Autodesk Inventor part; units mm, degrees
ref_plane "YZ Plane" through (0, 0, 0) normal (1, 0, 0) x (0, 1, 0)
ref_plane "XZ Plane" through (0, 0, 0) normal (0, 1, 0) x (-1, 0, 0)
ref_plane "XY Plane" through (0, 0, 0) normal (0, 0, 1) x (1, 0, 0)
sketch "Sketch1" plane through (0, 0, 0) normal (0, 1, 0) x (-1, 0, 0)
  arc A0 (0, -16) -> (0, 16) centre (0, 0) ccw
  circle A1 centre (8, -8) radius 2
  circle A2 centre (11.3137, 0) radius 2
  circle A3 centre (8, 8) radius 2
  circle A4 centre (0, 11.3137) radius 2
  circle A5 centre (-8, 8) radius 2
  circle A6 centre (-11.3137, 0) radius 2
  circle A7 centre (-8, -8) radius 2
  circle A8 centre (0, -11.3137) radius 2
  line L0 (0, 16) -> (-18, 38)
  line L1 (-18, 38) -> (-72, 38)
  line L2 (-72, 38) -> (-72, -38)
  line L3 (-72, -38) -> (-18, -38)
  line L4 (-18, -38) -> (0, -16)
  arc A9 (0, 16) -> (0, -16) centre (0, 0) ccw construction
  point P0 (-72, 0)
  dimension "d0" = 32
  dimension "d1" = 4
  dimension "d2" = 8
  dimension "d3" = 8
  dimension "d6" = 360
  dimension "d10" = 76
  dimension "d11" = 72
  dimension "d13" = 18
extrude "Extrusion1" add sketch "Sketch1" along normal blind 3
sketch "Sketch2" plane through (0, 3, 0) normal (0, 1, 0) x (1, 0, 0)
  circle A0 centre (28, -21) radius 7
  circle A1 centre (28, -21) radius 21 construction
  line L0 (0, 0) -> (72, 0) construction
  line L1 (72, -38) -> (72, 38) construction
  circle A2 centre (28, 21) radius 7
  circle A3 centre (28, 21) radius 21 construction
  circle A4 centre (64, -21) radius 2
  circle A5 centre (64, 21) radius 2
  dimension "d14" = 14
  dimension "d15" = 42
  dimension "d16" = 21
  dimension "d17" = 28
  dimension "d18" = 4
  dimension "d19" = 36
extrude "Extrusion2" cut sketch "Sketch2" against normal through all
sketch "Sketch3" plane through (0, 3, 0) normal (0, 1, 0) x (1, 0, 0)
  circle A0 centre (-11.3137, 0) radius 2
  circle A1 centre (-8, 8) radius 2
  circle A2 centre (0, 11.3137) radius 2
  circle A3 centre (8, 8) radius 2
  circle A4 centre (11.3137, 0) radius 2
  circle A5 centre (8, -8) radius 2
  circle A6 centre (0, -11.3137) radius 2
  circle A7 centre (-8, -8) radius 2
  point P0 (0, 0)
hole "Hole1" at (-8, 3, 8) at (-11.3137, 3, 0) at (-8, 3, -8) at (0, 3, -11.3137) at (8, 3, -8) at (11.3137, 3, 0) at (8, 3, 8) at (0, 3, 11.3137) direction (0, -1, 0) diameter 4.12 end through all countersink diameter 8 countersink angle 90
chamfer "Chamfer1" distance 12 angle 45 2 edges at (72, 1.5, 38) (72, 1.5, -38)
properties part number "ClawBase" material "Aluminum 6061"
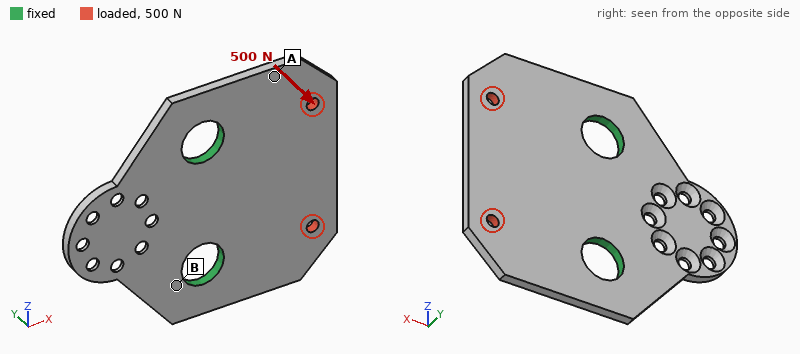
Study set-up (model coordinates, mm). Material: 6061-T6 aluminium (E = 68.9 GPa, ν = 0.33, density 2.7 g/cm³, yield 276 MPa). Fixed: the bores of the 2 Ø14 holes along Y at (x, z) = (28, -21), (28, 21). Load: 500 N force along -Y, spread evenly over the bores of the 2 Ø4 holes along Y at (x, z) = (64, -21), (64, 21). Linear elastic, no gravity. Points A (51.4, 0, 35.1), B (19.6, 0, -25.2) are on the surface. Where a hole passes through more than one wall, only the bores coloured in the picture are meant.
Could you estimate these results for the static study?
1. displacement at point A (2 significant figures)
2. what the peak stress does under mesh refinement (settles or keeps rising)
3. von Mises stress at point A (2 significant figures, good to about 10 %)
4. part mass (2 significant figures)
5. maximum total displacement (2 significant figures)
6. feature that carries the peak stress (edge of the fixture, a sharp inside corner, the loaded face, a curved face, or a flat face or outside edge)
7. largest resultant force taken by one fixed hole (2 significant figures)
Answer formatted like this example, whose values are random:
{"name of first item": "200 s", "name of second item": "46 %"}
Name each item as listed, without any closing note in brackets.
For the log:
{"displacement at point A": "0.16 mm", "what the peak stress does under mesh refinement": "keeps rising", "von Mises stress at point A": "57 MPa", "part mass": "39 g", "maximum total displacement": "0.57 mm", "feature that carries the peak stress": "edge of the fixture", "largest resultant force taken by one fixed hole": "250 N"}
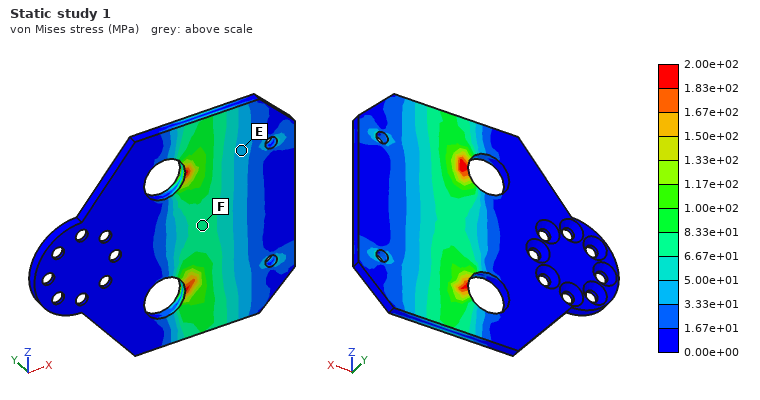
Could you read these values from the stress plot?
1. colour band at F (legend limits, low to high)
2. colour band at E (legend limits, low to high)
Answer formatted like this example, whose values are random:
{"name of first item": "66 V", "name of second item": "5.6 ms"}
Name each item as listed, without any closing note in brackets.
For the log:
{"colour band at F": "6.67e+01 to 8.33e+01 MPa", "colour band at E": "3.33e+01 to 5.00e+01 MPa"}
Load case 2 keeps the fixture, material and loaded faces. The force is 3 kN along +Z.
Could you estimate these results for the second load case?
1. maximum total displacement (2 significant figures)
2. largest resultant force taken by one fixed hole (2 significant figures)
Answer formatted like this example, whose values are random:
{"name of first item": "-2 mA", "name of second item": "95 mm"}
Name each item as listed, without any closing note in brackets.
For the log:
{"maximum total displacement": "31 µm", "largest resultant force taken by one fixed hole": "2.4 kN"}
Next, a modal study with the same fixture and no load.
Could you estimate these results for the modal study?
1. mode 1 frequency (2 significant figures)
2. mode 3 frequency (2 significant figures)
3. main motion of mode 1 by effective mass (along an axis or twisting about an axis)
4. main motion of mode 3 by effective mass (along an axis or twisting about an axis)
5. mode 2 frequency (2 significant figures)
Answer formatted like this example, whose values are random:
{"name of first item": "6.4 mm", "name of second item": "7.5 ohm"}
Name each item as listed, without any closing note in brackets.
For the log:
{"mode 1 frequency": "1800 Hz", "mode 3 frequency": "3000 Hz", "main motion of mode 1 by effective mass": "along Y", "main motion of mode 3 by effective mass": "twisting about X", "mode 2 frequency": "2400 Hz"}
